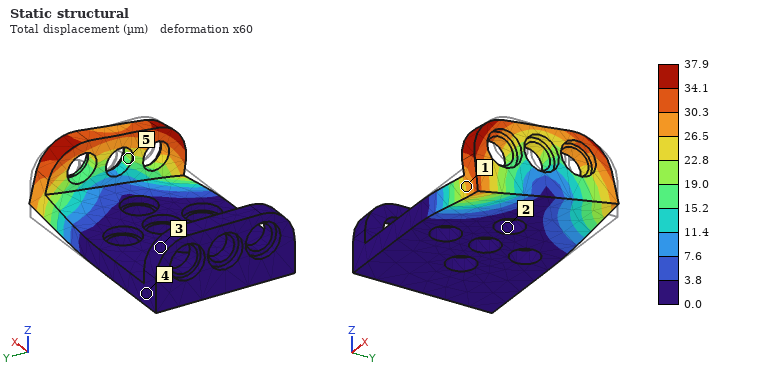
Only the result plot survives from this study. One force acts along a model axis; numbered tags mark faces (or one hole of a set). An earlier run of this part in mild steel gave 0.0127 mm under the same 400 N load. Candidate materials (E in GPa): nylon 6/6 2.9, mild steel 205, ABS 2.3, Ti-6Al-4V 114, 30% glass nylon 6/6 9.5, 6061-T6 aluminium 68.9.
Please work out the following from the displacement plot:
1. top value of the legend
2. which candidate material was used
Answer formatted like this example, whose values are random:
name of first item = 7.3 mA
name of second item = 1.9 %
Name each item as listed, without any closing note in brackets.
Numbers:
top value of the legend = 37.9 µm
which candidate material was used = 6061-T6 aluminium
